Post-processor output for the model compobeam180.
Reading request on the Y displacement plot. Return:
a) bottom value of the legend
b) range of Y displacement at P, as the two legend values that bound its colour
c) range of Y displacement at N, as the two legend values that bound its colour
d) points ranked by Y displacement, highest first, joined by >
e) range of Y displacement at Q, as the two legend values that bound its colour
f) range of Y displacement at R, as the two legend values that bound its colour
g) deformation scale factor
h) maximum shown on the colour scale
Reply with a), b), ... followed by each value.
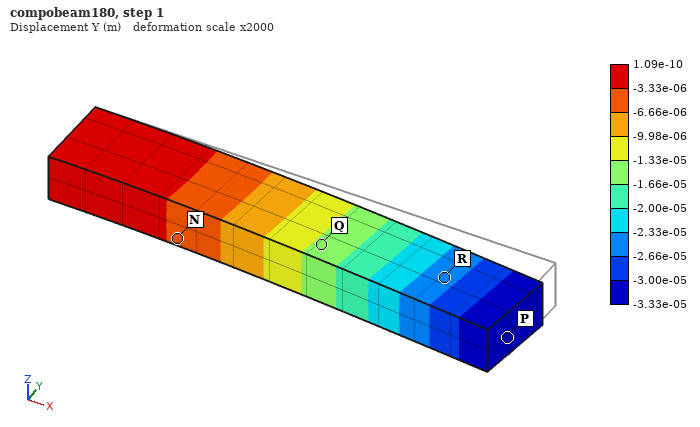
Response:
a) -3.33e-05 m
b) -3.33e-05 to -3.00e-05 m
c) -6.66e-06 to -3.33e-06 m
d) N > Q > R > P
e) -1.66e-05 to -1.33e-05 m
f) -2.66e-05 to -2.33e-05 m
g) 2000
h) 1.09e-10 m
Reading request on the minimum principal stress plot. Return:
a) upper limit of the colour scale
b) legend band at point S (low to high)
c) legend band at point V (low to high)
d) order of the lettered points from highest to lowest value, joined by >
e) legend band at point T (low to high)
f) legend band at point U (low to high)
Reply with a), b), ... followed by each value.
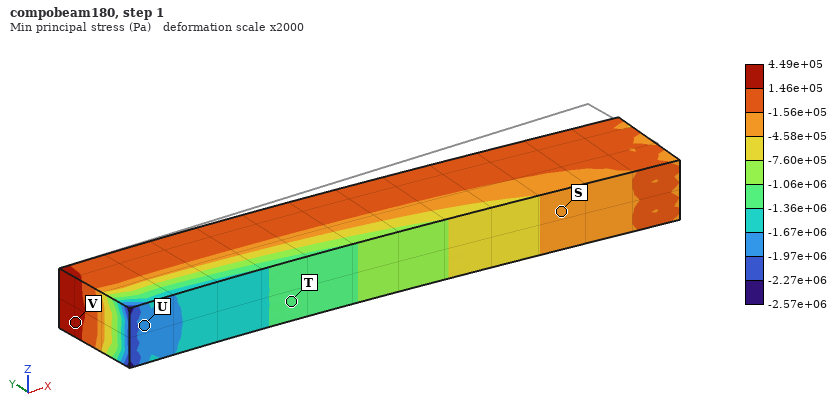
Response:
a) 4.49e+05 Pa
b) -4.58e+05 to -1.56e+05 Pa
c) 1.46e+05 to 4.49e+05 Pa
d) V > S > T > U
e) -1.36e+06 to -1.06e+06 Pa
f) -1.97e+06 to -1.67e+06 Pa
